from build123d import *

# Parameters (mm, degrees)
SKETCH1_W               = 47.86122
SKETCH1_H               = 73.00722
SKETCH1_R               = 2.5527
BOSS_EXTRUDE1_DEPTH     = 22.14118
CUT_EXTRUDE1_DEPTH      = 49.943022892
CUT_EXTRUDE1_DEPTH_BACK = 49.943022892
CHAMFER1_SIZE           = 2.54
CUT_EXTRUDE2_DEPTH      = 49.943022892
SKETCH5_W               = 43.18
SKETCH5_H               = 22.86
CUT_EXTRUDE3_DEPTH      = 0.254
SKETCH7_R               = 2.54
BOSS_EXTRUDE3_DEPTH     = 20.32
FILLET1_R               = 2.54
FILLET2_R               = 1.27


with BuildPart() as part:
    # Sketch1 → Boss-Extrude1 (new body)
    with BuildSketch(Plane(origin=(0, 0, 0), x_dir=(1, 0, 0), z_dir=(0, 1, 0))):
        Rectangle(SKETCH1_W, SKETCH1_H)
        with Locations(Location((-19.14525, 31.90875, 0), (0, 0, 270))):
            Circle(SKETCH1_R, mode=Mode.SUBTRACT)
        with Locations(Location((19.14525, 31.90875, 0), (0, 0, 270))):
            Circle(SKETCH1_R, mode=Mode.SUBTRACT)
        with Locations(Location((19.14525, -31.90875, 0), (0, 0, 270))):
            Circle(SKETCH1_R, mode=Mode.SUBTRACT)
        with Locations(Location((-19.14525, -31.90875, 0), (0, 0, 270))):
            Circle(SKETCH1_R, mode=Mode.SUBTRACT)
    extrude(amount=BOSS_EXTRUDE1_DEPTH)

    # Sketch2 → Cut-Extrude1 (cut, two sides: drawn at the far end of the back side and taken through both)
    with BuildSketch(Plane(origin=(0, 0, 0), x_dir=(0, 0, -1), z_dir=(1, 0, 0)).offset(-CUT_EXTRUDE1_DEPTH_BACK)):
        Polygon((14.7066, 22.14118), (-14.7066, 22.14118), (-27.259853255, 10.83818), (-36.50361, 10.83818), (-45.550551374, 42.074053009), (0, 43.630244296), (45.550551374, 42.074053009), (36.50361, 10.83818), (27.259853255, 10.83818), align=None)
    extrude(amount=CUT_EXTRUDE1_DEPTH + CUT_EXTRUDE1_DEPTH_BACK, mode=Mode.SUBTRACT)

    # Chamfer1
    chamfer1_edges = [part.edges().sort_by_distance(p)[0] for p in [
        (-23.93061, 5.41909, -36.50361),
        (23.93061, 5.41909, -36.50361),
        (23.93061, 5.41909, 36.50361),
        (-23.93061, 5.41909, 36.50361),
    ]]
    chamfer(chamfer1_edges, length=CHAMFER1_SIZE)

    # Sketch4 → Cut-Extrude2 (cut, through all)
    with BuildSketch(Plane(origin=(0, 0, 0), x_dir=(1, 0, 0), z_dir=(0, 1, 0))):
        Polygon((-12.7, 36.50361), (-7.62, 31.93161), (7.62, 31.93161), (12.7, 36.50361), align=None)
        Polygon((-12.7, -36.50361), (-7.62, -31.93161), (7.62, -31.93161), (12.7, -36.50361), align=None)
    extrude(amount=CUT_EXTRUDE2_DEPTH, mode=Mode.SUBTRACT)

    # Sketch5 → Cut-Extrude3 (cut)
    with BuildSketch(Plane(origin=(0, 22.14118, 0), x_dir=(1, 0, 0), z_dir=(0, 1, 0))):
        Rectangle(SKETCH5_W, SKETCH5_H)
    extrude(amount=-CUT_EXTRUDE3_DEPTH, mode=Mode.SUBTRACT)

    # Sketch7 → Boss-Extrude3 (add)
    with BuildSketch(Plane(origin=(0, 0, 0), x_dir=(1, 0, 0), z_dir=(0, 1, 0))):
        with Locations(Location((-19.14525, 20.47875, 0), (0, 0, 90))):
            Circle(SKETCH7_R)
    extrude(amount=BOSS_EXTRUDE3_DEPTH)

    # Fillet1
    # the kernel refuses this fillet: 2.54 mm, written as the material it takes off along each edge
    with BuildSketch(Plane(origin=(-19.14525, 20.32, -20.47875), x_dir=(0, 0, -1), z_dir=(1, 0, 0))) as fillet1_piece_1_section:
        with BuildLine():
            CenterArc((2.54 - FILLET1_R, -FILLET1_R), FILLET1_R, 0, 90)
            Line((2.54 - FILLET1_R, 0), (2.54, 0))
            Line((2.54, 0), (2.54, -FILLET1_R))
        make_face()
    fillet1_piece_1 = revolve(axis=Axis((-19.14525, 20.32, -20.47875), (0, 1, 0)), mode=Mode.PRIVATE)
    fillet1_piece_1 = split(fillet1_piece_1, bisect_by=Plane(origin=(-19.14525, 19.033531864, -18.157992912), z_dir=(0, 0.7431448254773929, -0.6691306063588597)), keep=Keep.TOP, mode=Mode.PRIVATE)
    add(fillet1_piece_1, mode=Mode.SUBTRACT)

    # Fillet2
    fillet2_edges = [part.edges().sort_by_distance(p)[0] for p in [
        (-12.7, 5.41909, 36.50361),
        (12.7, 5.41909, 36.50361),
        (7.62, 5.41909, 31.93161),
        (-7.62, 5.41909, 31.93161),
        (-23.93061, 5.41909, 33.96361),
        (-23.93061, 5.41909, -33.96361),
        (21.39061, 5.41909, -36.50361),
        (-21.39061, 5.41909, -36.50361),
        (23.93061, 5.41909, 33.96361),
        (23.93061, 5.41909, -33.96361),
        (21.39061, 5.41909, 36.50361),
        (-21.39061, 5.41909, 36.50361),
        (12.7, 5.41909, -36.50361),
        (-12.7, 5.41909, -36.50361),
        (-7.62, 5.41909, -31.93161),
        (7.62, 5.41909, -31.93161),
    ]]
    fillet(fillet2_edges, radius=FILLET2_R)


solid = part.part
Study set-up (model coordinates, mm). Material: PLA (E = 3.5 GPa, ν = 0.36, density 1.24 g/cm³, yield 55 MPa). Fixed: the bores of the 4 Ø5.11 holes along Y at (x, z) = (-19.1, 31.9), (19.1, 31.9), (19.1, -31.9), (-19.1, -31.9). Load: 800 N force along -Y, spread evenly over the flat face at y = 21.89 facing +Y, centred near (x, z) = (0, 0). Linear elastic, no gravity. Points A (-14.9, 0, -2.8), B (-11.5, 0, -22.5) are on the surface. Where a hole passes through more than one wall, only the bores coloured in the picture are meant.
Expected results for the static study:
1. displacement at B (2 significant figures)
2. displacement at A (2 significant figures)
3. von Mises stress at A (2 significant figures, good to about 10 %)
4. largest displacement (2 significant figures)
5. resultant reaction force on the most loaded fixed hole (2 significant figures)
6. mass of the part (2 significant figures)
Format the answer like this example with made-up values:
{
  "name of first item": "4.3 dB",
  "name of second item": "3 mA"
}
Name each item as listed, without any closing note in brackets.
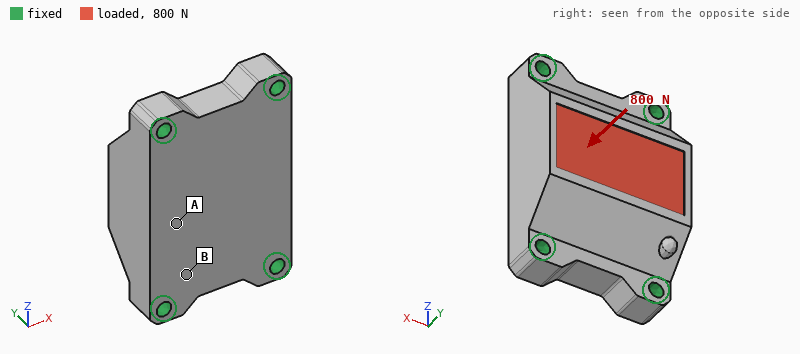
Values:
{
  "displacement at B": "16 µm",
  "displacement at A": "27 µm",
  "von Mises stress at A": "1.5 MPa",
  "largest displacement": "29 µm",
  "resultant reaction force on the most loaded fixed hole": "240 N",
  "mass of the part": "71 g"
}
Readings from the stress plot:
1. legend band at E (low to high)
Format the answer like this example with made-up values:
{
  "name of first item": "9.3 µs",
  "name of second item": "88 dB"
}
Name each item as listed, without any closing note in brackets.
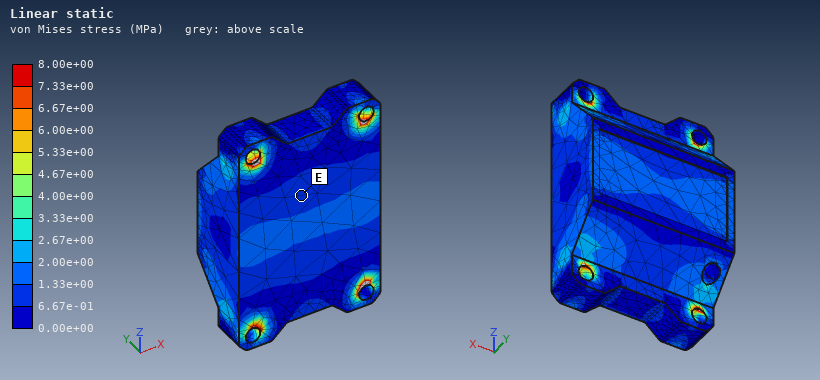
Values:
{
  "legend band at E": "6.67e-01 to 1.33e+00 MPa"
}
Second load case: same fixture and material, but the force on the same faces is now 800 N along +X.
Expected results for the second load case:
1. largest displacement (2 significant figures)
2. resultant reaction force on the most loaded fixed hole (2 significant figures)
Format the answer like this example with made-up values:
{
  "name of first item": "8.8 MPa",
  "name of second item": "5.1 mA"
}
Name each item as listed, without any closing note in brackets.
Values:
{
  "largest displacement": "46 µm",
  "resultant reaction force on the most loaded fixed hole": "320 N"
}
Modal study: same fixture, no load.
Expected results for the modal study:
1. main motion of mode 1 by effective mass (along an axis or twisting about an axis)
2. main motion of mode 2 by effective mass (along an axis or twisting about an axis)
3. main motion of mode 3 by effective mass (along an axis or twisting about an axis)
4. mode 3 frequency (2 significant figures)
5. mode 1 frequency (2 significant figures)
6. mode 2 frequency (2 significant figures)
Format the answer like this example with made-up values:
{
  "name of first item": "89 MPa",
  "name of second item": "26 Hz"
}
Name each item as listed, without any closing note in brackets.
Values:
{
  "main motion of mode 1 by effective mass": "along Y",
  "main motion of mode 2 by effective mass": "along X",
  "main motion of mode 3 by effective mass": "along X",
  "mode 3 frequency": "5700 Hz",
  "mode 1 frequency": "3900 Hz",
  "mode 2 frequency": "4600 Hz"
}
